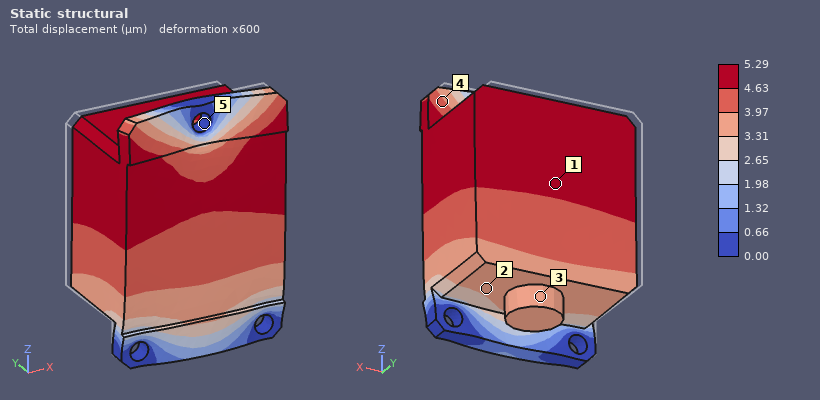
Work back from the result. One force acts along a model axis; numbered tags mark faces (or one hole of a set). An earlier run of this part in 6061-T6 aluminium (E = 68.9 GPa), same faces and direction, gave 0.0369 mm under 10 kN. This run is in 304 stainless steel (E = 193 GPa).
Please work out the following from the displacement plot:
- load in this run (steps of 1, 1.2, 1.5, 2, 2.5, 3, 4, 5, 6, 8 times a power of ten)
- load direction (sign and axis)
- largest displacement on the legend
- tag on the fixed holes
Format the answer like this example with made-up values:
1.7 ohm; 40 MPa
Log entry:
4 kN; -Y; 5.29 µm; 5
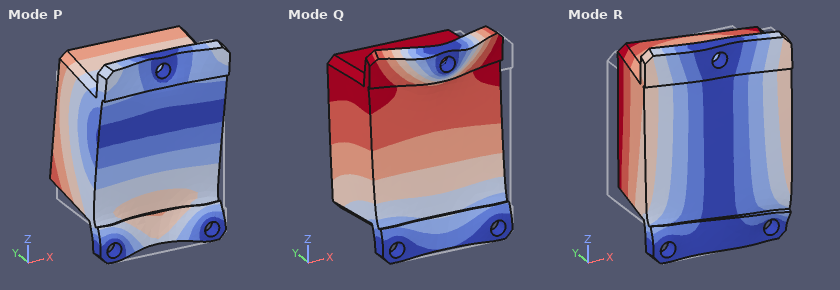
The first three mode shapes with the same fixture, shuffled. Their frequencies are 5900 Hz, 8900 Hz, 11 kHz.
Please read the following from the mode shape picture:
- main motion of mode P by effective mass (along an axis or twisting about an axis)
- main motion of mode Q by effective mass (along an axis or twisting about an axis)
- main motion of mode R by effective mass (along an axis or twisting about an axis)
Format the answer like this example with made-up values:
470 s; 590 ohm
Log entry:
along Z; along Y; along X
